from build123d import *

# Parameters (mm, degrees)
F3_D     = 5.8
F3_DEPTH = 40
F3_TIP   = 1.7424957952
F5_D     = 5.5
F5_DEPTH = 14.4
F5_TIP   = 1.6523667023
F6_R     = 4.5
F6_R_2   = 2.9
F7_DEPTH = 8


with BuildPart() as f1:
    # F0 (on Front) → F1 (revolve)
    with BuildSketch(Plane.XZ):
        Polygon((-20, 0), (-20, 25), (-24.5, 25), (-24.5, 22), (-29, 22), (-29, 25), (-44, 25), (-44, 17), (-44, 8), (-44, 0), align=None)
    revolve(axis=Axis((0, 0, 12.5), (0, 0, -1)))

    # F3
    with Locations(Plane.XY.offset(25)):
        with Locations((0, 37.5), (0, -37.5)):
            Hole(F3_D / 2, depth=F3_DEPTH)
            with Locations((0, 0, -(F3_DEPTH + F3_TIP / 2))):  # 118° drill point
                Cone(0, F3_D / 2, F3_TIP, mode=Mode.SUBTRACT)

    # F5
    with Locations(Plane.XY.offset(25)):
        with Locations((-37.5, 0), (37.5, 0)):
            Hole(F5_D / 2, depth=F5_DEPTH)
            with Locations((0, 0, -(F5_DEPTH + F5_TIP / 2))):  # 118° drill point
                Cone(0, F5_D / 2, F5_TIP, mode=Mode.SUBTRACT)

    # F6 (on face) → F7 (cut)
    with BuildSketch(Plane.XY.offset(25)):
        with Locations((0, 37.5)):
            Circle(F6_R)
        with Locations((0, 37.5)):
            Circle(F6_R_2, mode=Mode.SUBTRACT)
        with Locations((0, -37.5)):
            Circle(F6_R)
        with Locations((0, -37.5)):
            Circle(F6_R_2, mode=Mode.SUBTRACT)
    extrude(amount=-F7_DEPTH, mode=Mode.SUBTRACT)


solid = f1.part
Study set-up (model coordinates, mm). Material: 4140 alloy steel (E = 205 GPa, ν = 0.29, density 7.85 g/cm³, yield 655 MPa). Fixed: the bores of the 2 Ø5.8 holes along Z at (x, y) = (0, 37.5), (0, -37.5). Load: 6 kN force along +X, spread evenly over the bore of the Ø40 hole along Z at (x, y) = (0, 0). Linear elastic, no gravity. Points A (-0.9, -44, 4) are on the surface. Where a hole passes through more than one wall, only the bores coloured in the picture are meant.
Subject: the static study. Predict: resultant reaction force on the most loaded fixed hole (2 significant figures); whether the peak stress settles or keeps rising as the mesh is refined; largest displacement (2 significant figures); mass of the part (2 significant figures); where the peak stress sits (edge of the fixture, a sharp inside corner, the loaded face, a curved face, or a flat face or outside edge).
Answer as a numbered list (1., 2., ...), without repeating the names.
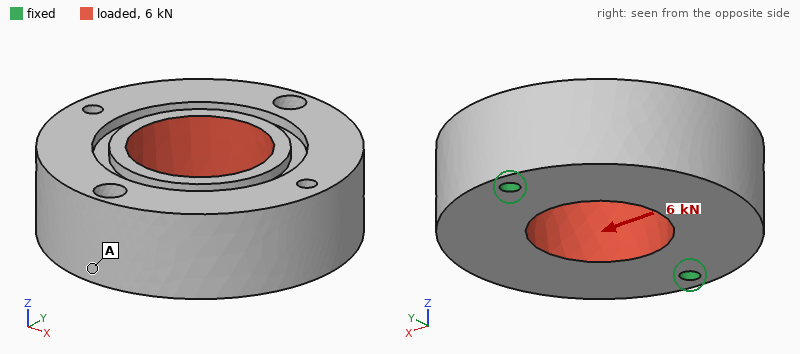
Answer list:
1. 3.0 kN
2. keeps rising
3. 2.3 µm
4. 910 g
5. edge of the fixture
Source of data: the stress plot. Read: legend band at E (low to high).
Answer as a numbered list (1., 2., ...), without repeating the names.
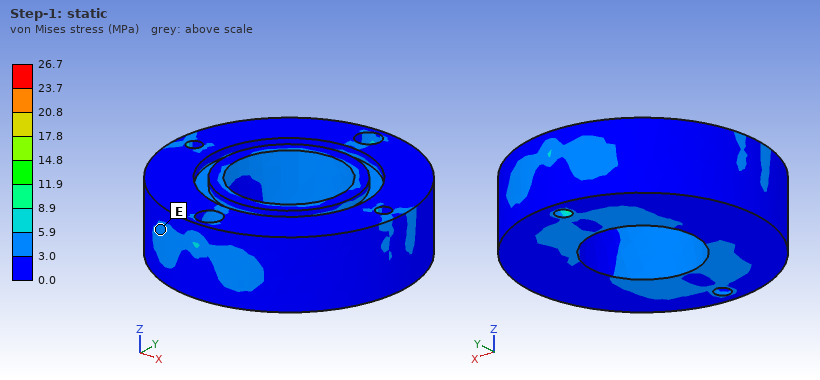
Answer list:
1. 3.0 to 5.9 MPa
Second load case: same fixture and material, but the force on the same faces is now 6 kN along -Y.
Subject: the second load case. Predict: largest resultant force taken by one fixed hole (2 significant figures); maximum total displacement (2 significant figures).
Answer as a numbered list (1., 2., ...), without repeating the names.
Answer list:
1. 3.0 kN
2. 1.3 µm
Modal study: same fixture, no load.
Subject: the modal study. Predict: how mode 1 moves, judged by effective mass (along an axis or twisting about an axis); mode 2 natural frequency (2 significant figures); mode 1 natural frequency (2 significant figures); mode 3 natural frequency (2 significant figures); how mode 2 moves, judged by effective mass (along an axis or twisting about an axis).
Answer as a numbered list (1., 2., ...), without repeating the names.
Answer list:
1. twisting about Y
2. 6600 Hz
3. 4600 Hz
4. 12 kHz
5. along Z
